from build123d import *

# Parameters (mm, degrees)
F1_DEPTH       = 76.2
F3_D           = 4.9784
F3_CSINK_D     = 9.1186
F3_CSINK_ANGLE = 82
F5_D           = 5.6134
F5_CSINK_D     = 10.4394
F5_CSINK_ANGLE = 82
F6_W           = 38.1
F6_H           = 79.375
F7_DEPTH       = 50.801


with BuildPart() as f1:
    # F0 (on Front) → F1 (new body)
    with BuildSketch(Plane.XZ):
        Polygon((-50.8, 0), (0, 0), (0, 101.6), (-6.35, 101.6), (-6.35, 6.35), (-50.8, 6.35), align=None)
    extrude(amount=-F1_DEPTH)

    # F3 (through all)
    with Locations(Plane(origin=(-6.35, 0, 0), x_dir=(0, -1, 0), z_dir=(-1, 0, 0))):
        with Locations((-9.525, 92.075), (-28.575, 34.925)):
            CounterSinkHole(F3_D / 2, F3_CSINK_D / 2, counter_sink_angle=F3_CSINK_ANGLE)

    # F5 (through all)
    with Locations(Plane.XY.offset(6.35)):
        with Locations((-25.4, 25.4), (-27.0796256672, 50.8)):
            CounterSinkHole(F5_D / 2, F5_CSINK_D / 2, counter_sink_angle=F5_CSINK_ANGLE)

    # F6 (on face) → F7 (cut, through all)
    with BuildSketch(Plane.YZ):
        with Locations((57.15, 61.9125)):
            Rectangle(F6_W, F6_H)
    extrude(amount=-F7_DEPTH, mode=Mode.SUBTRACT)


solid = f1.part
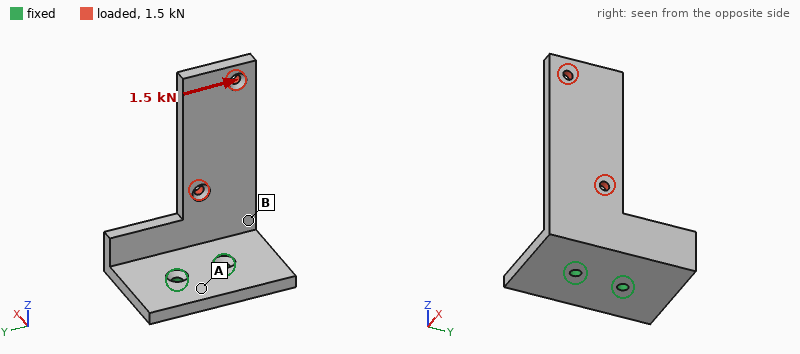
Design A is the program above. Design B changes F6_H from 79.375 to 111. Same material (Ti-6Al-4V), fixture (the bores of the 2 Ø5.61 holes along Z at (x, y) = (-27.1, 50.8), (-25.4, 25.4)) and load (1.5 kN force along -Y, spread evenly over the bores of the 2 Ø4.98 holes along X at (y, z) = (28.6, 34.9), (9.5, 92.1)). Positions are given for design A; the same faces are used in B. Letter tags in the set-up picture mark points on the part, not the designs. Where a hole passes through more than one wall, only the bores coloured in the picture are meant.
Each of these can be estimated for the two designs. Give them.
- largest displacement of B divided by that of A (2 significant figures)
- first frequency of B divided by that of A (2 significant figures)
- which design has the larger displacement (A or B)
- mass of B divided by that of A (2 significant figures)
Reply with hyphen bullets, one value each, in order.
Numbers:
- 1.8
- 0.94
- B
- 0.92
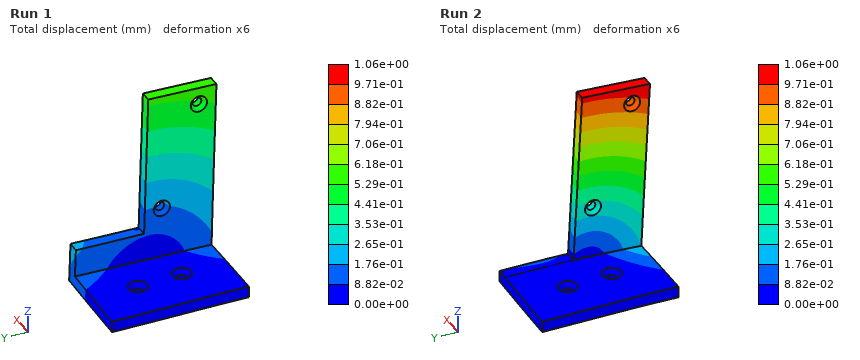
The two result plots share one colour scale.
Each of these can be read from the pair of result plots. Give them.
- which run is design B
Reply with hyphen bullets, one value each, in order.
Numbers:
- Run 2
